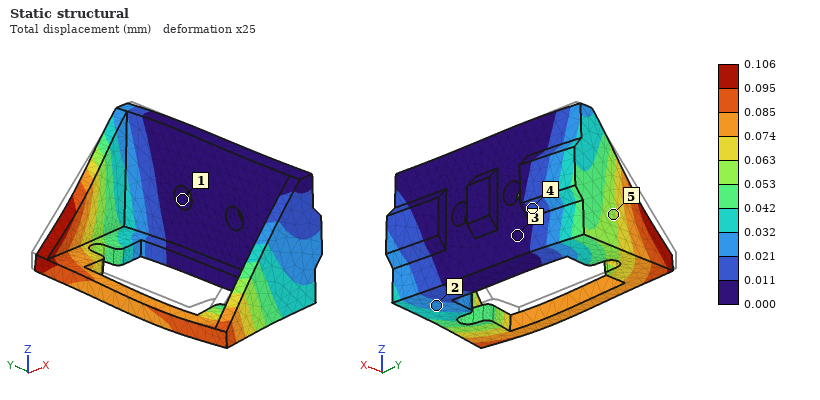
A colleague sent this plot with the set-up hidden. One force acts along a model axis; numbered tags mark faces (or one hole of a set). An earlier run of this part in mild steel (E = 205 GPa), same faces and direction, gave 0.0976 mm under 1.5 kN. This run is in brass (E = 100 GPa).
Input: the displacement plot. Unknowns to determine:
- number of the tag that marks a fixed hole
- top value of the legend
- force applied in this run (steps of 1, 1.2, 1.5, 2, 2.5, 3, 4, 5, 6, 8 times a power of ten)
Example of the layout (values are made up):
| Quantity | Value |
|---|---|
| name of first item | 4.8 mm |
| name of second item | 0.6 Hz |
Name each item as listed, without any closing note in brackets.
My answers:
| Quantity | Value |
|---|---|
| number of the tag that marks a fixed hole | 1 |
| top value of the legend | 0.106 mm |
| force applied in this run | 800 N |
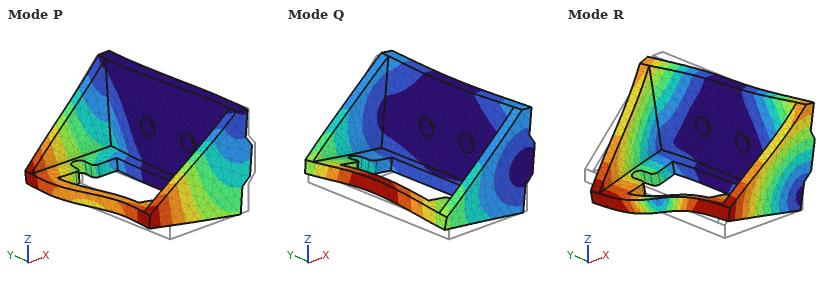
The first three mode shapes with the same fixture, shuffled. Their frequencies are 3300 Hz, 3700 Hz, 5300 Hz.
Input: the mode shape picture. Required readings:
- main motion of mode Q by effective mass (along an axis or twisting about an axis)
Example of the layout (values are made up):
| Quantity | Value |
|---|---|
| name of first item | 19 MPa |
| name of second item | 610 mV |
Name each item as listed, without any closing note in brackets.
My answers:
| Quantity | Value |
|---|---|
| main motion of mode Q by effective mass | along Z |
